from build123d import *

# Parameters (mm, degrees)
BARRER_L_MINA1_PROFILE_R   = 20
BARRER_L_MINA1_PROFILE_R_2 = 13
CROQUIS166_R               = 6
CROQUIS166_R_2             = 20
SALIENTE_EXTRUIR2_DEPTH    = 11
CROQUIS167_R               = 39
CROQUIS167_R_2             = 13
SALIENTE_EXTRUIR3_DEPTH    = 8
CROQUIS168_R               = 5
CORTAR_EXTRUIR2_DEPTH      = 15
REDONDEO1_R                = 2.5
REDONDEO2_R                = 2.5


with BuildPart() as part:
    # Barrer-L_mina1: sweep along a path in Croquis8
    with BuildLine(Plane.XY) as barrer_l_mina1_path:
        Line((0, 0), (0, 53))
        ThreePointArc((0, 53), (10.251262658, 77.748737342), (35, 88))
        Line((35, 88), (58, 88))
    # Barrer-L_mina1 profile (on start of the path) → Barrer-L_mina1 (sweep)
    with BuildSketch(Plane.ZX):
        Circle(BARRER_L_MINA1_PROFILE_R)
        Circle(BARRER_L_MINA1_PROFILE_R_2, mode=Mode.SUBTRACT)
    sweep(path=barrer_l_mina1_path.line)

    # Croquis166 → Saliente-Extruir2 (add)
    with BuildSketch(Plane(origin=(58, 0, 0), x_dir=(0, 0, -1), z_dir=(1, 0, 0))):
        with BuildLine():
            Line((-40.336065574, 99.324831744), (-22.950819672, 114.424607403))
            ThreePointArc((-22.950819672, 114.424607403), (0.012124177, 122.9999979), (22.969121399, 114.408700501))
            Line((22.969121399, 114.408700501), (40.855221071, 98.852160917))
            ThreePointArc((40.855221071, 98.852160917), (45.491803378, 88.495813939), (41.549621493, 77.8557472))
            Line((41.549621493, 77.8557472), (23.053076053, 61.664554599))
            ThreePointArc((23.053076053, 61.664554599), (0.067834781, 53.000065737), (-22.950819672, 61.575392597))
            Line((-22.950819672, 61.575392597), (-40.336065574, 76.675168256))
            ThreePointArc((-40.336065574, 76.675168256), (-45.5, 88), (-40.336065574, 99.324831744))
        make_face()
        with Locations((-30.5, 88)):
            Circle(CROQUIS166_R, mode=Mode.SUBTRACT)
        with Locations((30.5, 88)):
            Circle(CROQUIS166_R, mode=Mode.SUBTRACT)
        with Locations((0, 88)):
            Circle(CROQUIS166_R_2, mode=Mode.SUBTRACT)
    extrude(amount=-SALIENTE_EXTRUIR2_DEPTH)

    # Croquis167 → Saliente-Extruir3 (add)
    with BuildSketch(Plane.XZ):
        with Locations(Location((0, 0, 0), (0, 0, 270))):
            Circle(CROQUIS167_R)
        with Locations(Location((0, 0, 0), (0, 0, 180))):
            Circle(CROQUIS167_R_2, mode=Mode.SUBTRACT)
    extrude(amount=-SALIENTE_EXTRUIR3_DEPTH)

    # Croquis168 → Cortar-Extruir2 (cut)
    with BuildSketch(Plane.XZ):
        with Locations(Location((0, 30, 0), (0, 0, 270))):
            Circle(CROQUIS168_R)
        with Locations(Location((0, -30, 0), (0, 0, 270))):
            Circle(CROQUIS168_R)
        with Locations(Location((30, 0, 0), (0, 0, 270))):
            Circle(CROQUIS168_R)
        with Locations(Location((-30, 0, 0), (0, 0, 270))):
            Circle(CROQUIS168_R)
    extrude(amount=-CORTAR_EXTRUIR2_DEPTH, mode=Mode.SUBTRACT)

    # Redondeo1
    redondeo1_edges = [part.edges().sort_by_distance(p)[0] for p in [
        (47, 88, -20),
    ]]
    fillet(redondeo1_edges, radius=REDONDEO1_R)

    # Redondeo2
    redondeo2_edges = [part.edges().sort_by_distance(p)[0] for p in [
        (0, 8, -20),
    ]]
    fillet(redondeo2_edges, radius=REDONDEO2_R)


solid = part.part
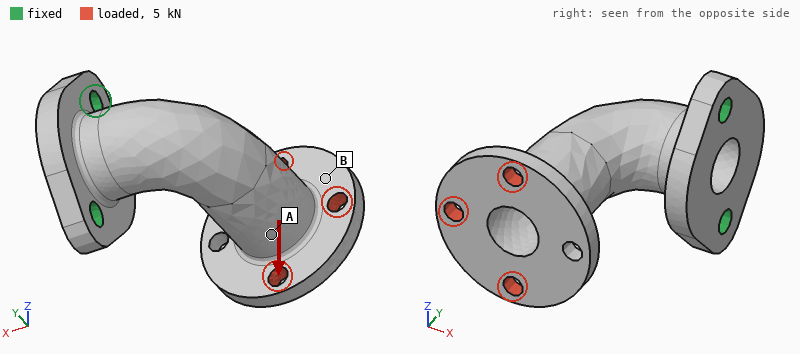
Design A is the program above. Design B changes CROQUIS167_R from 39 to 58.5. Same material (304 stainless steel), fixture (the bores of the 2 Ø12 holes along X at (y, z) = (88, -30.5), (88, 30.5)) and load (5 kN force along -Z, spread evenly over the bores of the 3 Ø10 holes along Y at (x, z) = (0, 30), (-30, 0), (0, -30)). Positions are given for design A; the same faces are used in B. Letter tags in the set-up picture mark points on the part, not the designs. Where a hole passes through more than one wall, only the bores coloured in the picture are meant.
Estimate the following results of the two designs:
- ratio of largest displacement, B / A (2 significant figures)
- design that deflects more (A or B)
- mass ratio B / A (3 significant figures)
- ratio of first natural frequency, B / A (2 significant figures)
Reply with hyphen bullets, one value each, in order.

- 1.1
- B
- 1.31
- 0.72
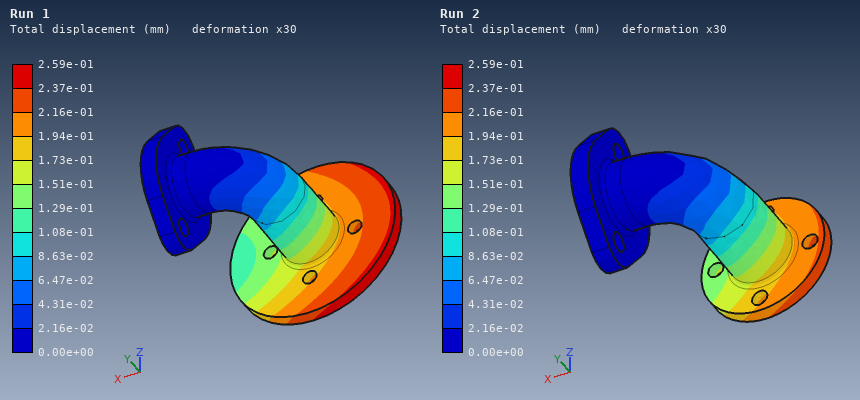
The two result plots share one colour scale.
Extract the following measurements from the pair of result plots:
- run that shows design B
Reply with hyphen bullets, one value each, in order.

- Run 1
